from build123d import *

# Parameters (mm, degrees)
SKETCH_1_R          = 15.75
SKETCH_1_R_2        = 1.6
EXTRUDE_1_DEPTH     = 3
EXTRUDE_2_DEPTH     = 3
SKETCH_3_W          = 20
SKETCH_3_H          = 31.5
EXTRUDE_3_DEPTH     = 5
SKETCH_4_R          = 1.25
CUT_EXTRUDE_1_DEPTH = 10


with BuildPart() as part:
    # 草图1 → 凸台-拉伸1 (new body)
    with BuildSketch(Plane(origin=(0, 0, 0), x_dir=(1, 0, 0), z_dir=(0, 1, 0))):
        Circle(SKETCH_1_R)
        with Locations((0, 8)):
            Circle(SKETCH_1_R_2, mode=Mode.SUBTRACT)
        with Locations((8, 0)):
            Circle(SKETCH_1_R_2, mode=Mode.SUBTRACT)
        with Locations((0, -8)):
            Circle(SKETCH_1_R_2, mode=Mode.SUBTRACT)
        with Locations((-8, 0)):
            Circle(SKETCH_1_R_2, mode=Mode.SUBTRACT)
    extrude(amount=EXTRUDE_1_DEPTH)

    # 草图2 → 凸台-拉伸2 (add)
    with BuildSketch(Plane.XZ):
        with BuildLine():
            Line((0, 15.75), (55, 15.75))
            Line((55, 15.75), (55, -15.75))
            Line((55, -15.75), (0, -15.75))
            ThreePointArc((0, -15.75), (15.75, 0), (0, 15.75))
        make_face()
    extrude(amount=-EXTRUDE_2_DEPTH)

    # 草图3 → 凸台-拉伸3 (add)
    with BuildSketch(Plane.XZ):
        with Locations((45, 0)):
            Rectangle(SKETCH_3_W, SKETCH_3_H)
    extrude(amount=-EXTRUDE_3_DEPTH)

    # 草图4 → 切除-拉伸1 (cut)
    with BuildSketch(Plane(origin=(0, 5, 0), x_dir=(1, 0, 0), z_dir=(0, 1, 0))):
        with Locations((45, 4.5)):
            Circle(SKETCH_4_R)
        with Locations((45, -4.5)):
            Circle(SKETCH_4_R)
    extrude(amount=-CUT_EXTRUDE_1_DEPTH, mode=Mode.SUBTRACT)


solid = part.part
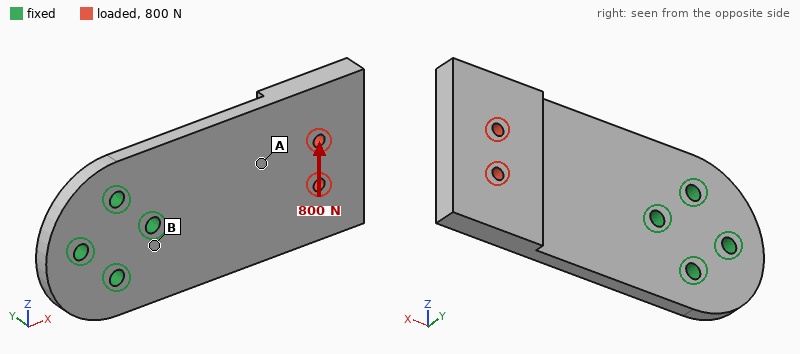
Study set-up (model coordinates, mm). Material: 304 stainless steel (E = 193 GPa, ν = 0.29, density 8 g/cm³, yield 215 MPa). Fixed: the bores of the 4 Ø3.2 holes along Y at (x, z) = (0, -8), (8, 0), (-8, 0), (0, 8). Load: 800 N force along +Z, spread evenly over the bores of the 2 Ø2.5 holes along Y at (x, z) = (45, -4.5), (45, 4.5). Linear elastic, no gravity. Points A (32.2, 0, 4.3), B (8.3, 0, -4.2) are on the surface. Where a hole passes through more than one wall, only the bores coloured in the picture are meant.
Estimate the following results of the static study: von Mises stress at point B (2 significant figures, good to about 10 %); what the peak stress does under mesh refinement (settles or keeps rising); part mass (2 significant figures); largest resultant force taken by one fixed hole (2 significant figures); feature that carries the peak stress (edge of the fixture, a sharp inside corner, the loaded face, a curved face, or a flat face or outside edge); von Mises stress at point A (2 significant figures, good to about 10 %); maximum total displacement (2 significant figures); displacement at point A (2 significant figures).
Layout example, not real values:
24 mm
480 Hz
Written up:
39 MPa
keeps rising
60 g
1.3 kN
edge of the fixture
14 MPa
34 µm
13 µm
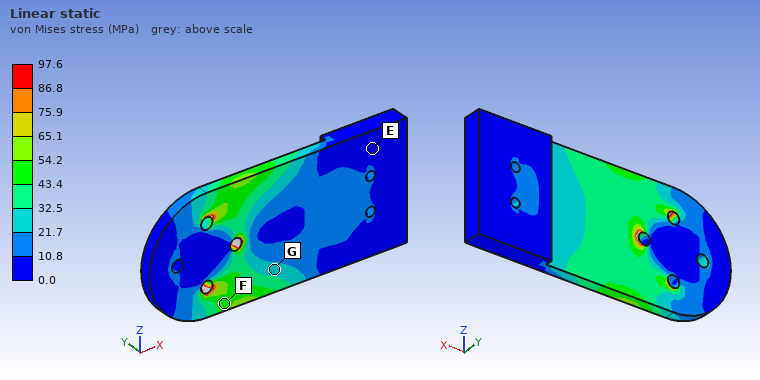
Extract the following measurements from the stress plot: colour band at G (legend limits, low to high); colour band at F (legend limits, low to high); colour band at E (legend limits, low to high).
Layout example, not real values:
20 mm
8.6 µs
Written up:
21.7 to 32.5 MPa
43.4 to 54.2 MPa
0.0 to 10.8 MPa
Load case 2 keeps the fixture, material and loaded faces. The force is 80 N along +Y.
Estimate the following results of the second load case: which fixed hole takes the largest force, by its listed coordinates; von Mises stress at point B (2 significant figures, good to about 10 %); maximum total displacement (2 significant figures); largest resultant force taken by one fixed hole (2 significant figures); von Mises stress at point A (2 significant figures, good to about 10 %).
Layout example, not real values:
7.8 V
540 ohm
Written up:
(8, 0)
41 MPa
0.14 mm
240 N
20 MPa
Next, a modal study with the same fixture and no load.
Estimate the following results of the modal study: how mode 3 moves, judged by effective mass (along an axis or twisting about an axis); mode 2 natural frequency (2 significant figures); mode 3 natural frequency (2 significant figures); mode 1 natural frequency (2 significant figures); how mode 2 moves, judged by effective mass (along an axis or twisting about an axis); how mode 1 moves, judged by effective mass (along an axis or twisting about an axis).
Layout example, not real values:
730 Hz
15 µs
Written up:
along Z
2700 Hz
5500 Hz
840 Hz
twisting about X
along Y
